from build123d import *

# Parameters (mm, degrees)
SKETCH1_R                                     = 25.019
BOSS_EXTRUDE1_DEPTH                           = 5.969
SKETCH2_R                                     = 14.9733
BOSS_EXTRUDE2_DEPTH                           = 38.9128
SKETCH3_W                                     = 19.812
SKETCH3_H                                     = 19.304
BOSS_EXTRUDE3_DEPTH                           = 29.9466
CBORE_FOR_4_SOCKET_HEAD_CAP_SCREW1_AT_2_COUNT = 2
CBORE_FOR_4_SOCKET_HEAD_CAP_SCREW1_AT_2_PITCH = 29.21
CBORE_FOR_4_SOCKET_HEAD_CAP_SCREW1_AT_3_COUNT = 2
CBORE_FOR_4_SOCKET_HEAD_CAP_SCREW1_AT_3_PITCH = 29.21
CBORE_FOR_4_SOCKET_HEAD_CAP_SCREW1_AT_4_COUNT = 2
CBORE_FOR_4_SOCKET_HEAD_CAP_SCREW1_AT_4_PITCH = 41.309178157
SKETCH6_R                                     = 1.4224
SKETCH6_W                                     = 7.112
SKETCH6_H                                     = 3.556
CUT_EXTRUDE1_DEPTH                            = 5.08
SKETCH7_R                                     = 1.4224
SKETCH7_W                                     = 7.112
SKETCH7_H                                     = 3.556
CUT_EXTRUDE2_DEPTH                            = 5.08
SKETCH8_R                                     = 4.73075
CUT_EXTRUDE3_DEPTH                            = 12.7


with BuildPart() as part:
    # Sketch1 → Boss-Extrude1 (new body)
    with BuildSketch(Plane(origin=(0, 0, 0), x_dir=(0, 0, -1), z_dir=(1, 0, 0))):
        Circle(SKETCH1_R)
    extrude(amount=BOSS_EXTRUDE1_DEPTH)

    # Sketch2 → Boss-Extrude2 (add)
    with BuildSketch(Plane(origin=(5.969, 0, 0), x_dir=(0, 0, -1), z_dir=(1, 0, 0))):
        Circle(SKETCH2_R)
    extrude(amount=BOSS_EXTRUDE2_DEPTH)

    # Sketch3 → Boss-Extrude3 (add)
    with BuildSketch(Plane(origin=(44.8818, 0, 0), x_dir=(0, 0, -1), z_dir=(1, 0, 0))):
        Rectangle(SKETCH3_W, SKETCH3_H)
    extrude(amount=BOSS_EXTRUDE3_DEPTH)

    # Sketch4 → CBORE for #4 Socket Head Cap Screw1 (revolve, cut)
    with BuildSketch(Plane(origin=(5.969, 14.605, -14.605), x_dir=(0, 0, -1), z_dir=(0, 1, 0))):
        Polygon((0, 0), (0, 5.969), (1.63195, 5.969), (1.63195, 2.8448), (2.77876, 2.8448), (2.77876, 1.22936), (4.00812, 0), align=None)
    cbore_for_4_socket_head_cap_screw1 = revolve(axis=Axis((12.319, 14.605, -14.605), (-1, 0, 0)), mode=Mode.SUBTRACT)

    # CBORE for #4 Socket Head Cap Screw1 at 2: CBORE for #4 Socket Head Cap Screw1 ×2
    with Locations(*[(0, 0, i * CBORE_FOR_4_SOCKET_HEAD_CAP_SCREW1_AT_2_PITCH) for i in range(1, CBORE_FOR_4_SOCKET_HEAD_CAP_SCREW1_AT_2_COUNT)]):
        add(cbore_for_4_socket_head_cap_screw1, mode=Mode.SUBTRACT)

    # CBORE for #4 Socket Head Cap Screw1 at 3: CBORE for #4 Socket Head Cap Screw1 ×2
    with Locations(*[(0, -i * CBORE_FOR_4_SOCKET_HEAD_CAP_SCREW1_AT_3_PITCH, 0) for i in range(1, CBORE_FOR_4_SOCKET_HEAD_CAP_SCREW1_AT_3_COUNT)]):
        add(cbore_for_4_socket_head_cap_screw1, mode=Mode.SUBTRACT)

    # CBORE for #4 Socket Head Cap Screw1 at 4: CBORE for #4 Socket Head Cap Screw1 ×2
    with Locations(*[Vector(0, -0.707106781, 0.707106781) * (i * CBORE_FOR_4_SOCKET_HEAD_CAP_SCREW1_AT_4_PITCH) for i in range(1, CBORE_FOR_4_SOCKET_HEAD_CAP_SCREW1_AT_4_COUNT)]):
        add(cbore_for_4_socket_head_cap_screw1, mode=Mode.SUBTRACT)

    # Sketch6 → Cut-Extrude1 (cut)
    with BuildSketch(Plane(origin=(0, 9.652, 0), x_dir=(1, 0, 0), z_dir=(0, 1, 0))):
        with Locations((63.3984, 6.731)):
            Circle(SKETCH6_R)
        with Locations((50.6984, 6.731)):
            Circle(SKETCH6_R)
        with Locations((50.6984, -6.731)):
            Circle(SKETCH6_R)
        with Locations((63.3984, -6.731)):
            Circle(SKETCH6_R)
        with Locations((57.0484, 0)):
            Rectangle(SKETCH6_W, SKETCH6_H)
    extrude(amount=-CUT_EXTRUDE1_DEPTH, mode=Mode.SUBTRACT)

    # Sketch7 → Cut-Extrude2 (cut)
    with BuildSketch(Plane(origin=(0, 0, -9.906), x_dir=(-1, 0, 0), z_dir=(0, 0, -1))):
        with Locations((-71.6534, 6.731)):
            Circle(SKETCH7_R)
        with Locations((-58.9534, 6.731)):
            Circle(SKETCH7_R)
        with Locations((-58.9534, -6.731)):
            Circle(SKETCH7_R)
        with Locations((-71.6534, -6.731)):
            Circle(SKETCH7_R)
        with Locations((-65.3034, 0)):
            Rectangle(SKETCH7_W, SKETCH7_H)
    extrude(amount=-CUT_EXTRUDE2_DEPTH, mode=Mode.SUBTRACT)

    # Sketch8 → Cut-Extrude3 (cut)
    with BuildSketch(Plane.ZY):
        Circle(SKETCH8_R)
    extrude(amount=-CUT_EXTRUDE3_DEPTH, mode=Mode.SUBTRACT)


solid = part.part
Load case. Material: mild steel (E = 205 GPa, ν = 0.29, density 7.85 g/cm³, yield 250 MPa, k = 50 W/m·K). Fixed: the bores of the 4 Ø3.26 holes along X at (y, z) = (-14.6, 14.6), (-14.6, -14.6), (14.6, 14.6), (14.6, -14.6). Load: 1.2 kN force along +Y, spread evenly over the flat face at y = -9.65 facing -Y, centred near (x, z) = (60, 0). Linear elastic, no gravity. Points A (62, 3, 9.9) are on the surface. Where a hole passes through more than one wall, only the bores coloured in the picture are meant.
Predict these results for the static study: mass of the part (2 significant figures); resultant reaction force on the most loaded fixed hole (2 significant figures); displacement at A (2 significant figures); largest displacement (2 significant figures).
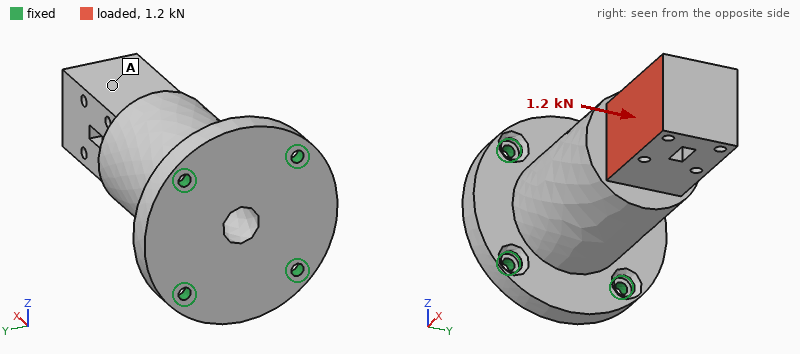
380 g
1.4 kN
28 µm
36 µm
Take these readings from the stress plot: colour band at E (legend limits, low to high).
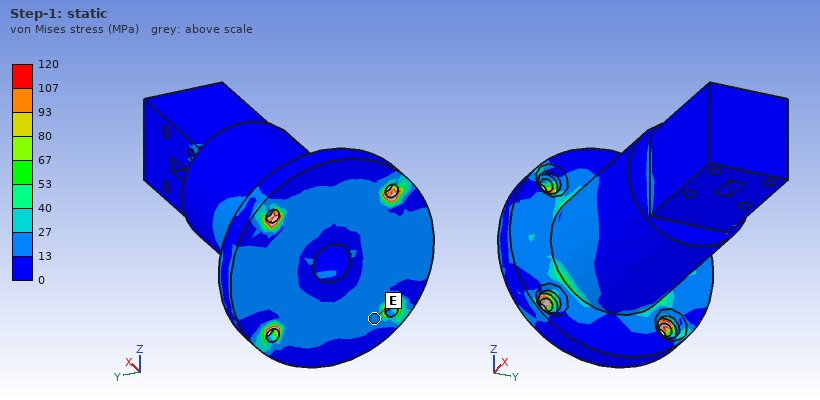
13 to 27 MPa
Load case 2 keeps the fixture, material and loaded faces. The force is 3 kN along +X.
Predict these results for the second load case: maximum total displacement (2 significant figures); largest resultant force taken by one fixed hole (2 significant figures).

23 µm
1.4 kN
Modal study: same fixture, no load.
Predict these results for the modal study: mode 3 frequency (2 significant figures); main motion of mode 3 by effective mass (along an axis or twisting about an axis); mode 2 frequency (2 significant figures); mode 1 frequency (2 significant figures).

9100 Hz
along X
3000 Hz
3000 Hz
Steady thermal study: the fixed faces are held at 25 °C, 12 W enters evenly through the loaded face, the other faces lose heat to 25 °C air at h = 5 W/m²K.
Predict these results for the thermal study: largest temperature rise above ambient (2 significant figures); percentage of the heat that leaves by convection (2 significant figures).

33 K
6.2 %
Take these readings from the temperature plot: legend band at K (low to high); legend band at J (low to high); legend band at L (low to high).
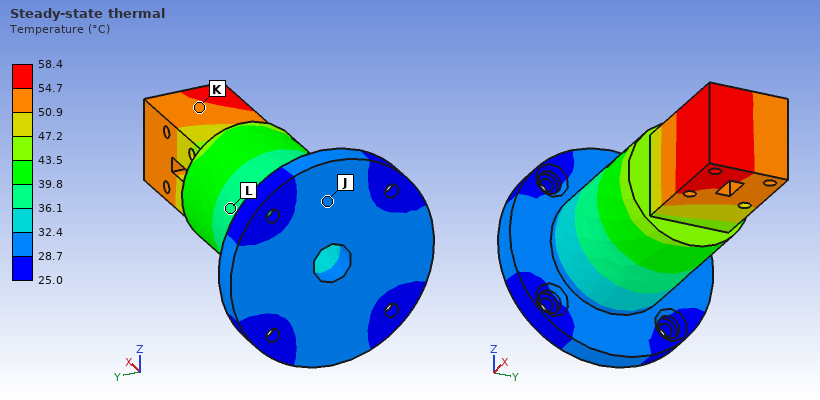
50.9 to 54.7 °C
28.7 to 32.4 °C
36.1 to 39.8 °C
